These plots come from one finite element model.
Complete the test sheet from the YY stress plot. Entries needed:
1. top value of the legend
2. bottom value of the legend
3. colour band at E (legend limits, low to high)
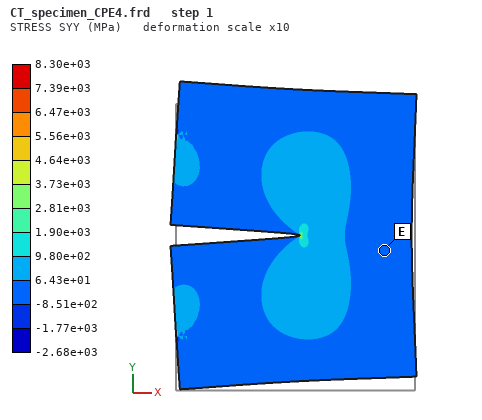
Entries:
8.30e+03 MPa
-2.68e+03 MPa
-8.51e+02 to 6.43e+01 MPa
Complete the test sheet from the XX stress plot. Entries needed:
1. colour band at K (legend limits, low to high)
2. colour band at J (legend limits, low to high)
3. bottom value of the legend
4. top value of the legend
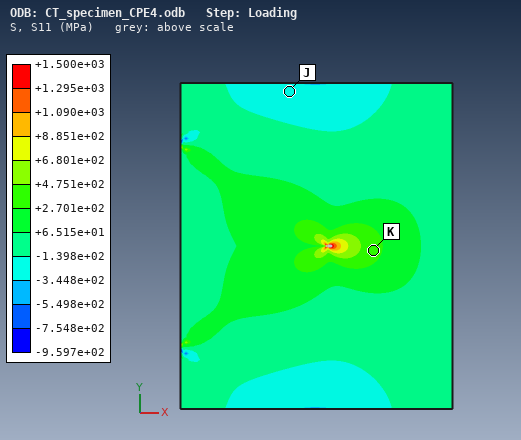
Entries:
+2.701e+02 to +4.751e+02 MPa
-3.448e+02 to -1.398e+02 MPa
-9.597e+02 MPa
+1.500e+03 MPa
